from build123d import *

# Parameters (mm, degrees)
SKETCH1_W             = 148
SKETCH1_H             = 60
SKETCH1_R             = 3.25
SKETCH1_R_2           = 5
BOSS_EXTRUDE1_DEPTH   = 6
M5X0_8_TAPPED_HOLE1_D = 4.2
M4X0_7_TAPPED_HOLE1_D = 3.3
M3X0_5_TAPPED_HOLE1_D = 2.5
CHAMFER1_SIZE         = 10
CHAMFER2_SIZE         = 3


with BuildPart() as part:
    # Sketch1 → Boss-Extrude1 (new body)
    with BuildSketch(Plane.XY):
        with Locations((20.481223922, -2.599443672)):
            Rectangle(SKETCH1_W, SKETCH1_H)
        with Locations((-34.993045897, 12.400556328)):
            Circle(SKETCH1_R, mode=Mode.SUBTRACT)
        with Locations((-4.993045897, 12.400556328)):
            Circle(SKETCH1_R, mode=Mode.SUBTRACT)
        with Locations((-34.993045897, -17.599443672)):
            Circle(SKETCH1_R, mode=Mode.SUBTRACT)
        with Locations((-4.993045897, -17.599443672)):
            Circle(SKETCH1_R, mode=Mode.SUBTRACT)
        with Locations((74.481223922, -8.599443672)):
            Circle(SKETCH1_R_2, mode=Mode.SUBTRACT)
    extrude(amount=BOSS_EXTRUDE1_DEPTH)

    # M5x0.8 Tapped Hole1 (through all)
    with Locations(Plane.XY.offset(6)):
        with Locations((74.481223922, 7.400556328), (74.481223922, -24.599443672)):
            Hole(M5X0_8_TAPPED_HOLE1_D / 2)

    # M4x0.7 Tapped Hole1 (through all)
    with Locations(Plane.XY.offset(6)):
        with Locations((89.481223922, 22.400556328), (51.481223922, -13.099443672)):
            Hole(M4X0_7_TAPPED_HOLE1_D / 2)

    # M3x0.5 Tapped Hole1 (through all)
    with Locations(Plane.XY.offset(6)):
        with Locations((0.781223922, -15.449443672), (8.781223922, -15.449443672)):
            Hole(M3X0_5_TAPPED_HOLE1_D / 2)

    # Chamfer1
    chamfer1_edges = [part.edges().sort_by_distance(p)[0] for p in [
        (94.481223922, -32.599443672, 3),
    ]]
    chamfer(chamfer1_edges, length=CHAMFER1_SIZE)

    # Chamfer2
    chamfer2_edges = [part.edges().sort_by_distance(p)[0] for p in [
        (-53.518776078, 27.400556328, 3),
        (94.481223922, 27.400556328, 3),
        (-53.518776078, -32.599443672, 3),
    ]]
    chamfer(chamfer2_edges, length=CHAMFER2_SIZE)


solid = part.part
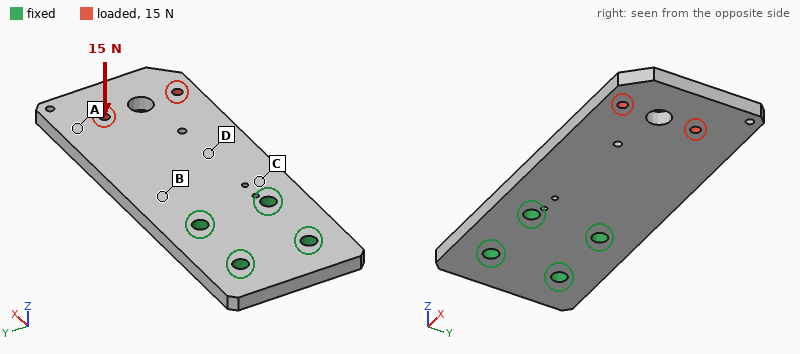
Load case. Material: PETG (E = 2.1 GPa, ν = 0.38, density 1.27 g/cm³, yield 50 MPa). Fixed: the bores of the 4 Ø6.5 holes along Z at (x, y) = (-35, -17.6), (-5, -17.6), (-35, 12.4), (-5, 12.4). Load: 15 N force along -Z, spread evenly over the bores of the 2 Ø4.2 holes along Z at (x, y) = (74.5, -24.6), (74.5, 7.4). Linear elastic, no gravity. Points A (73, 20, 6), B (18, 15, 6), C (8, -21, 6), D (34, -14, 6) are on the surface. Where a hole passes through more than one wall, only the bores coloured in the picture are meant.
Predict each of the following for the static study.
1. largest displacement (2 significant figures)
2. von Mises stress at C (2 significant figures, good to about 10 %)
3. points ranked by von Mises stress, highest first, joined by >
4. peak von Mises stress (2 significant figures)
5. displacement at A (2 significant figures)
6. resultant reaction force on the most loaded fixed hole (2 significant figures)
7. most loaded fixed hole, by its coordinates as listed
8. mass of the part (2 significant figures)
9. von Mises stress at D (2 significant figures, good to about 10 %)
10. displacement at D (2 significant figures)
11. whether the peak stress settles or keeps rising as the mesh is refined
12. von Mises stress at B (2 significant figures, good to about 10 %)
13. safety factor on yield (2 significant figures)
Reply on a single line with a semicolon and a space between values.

1.5 mm; 2.8 MPa; C > B > D > A; 9.3 MPa; 0.99 mm; 13 N; (-5, -17.6); 65 g; 1.6 MPa; 0.33 mm; settles; 2.2 MPa; 5.4
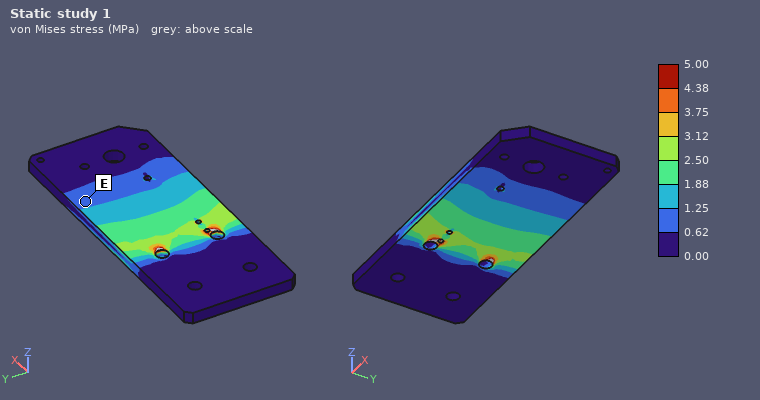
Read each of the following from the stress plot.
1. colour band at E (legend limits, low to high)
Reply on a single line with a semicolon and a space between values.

0.62 to 1.25 MPa
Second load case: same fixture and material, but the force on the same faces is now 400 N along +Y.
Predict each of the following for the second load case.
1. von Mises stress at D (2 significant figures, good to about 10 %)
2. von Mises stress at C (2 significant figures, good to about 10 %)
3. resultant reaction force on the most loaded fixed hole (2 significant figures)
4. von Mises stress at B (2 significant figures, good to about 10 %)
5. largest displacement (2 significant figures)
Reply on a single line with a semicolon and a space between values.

3.1 MPa; 5.8 MPa; 730 N; 4.3 MPa; 0.69 mm
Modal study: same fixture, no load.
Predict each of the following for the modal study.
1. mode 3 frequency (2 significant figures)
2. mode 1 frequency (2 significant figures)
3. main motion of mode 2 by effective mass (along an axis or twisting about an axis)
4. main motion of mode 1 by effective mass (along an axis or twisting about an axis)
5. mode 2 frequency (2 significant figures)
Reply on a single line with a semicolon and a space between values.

790 Hz; 130 Hz; twisting about X; along Z; 450 Hz
